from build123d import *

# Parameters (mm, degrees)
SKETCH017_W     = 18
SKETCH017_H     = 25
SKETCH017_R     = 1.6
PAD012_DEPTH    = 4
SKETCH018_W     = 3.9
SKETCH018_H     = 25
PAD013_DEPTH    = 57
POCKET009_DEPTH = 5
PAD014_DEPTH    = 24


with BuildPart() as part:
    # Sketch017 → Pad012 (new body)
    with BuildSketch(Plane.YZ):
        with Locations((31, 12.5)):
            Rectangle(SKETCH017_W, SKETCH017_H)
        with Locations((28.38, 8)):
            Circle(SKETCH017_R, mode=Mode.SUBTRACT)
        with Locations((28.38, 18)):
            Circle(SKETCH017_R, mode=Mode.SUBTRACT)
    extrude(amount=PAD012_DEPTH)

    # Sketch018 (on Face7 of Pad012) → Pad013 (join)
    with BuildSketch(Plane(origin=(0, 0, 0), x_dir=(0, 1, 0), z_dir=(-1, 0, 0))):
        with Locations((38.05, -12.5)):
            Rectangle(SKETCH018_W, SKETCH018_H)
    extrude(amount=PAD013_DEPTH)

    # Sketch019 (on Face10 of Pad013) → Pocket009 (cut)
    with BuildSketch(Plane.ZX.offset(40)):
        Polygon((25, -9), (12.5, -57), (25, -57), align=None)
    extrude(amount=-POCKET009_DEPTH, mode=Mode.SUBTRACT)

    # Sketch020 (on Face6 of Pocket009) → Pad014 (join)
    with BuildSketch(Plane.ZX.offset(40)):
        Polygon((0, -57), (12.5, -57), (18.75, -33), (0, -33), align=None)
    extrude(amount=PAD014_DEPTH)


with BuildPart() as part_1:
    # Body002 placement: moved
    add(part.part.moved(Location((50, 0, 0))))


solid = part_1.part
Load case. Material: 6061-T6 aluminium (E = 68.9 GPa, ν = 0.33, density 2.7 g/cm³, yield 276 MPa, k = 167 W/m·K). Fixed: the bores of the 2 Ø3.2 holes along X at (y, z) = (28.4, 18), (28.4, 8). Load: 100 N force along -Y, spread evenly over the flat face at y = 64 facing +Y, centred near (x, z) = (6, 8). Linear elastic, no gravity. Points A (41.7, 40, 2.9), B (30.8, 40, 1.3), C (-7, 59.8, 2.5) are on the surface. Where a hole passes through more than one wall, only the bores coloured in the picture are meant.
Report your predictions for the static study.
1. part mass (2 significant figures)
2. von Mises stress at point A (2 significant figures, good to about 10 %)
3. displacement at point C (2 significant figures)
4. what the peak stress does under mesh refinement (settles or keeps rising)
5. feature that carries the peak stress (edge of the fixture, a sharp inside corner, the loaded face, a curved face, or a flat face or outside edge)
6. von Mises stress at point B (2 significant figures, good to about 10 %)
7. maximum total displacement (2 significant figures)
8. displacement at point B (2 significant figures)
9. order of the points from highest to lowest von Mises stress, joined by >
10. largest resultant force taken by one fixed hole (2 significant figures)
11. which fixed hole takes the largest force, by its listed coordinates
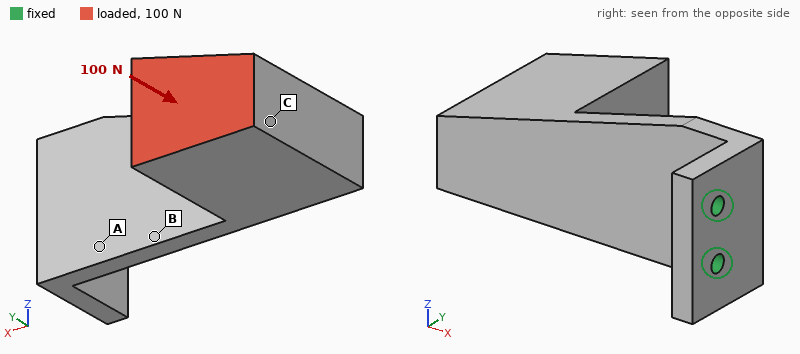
41 g
59 MPa
0.88 mm
keeps rising
edge of the fixture
44 MPa
0.92 mm
0.20 mm
A > B > C
100 N
(28.4, 8)
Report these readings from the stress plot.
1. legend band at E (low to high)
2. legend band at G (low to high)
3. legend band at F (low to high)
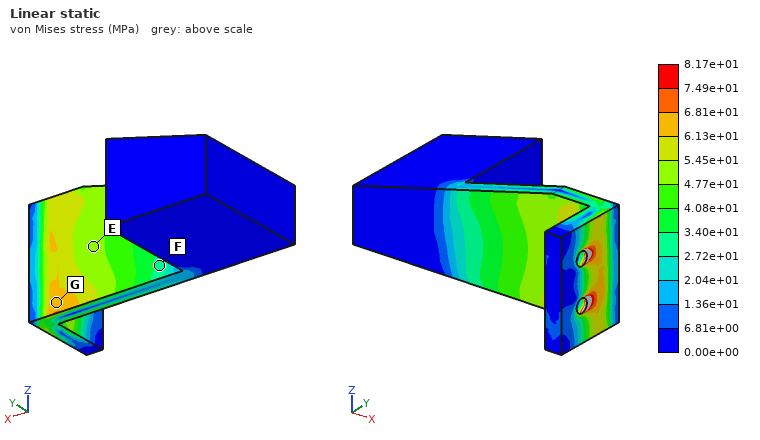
4.77e+01 to 5.45e+01 MPa
6.13e+01 to 6.81e+01 MPa
2.72e+01 to 3.40e+01 MPa
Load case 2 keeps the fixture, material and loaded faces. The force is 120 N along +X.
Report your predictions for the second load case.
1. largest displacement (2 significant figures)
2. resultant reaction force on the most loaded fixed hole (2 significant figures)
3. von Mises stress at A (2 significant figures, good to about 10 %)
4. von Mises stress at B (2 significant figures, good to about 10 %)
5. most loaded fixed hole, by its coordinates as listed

0.92 mm
100 N
53 MPa
59 MPa
(28.4, 8)
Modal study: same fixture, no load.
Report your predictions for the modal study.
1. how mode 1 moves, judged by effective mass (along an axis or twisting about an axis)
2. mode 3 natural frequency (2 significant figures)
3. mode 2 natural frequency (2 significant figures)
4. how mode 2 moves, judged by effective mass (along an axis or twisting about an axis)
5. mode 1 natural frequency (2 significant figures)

along Y
2000 Hz
890 Hz
along Z
350 Hz
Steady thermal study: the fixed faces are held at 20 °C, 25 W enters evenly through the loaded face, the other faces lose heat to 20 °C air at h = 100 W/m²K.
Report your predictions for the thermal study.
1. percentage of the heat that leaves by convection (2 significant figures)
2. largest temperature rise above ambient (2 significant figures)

57 %
48 K
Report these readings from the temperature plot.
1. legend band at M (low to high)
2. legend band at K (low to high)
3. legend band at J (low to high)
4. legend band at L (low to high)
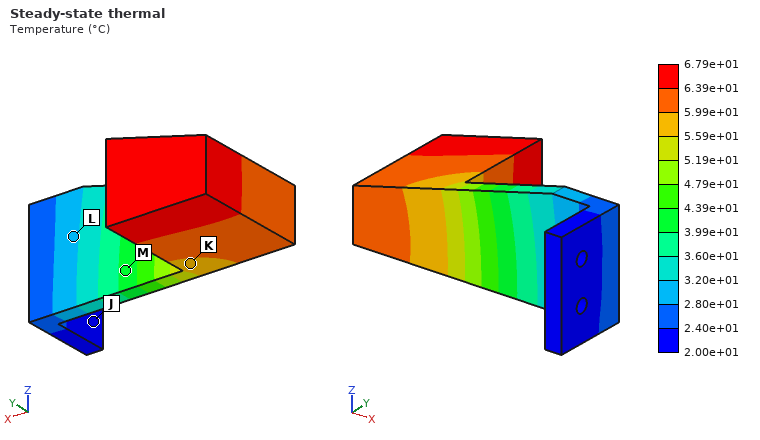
3.99e+01 to 4.39e+01 °C
5.59e+01 to 5.99e+01 °C
2.00e+01 to 2.40e+01 °C
2.80e+01 to 3.20e+01 °C
